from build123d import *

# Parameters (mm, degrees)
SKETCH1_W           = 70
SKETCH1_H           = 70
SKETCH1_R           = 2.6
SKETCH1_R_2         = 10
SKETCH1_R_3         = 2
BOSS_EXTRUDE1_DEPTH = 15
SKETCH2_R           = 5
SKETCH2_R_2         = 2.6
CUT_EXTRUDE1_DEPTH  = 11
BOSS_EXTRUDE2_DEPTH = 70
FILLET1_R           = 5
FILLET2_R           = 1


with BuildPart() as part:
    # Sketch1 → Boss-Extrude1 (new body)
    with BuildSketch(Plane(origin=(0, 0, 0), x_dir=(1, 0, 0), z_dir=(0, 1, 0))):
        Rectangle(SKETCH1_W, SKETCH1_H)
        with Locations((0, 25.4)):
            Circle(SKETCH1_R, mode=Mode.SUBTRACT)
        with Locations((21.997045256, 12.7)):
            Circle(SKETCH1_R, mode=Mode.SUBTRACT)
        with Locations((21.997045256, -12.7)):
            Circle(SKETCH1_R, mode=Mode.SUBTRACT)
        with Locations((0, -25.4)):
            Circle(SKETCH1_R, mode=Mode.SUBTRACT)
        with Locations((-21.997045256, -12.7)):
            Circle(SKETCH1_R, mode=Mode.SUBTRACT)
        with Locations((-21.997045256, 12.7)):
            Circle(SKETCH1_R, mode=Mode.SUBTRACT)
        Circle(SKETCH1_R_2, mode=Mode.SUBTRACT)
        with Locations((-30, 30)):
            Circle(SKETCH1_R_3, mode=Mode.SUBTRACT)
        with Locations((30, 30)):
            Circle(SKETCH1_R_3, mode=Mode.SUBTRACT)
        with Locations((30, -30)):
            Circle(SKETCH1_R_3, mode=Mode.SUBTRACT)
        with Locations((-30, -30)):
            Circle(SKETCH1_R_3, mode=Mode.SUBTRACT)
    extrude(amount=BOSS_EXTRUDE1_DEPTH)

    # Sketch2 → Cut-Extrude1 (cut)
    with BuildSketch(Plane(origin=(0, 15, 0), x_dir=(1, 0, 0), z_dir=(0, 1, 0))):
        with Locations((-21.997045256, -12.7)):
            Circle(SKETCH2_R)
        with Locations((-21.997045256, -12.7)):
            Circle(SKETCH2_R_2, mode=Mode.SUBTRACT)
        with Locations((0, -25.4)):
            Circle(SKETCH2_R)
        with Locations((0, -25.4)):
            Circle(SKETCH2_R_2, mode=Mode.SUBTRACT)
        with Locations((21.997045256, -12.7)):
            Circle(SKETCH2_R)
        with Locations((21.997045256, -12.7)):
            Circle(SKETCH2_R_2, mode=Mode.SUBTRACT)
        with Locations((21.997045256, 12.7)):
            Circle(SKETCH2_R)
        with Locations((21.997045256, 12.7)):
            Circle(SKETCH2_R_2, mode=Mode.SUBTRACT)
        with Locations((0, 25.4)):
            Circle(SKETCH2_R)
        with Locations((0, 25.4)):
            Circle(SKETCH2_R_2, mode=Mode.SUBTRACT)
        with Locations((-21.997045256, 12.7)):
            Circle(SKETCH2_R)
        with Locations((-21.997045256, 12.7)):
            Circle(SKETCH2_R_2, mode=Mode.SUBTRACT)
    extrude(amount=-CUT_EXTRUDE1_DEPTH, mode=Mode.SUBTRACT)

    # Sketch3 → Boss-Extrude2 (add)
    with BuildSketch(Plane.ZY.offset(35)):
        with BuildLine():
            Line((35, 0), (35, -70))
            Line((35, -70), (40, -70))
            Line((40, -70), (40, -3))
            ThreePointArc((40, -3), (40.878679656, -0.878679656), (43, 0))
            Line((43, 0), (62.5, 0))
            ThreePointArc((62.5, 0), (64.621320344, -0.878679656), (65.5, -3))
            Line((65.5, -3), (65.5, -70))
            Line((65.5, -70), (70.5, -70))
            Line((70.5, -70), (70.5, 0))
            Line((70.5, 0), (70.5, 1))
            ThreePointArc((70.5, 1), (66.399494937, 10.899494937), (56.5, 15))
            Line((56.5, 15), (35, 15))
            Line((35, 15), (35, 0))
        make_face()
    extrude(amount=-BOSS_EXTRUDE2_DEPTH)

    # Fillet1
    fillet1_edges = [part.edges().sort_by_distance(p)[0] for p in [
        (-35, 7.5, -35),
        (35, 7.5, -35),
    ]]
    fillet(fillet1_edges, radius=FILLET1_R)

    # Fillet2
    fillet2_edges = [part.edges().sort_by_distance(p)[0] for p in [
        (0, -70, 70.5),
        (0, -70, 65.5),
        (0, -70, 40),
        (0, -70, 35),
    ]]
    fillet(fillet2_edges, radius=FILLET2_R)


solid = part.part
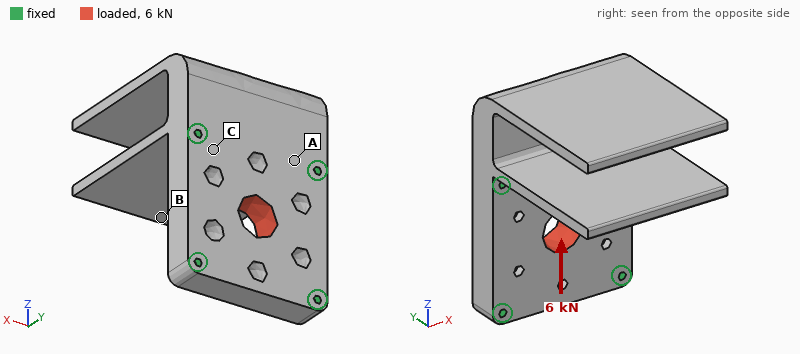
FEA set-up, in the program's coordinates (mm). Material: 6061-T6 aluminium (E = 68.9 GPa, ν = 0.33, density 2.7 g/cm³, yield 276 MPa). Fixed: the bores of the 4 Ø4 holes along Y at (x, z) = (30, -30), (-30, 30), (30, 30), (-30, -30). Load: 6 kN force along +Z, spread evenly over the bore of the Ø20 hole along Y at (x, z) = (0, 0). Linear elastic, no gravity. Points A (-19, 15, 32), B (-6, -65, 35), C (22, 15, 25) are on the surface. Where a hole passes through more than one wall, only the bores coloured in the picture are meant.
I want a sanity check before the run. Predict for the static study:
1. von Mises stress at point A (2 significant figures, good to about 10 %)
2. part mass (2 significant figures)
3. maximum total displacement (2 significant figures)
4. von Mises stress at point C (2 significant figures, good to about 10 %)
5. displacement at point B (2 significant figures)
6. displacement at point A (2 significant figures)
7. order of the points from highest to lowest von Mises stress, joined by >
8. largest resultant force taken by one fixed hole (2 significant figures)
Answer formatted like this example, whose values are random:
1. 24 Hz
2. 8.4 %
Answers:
1. 3.6 MPa
2. 390 g
3. 5.1 µm
4. 6.4 MPa
5. 2.8 µm
6. 1.5 µm
7. C > A > B
8. 1.8 kN
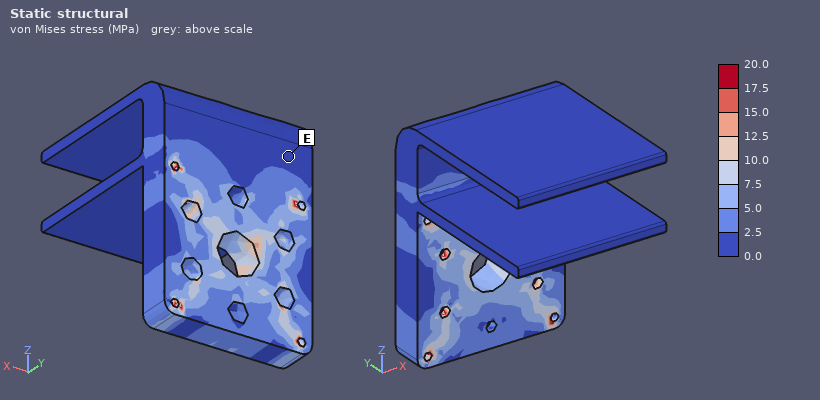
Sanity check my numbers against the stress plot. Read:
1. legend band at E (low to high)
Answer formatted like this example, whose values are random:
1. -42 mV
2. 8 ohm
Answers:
1. 0.0 to 2.5 MPa
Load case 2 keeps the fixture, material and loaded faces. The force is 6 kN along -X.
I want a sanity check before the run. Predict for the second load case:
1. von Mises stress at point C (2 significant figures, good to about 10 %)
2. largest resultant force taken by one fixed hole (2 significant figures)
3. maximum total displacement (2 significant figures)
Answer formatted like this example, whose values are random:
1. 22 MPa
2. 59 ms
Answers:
1. 9.4 MPa
2. 1.7 kN
3. 5.8 µm
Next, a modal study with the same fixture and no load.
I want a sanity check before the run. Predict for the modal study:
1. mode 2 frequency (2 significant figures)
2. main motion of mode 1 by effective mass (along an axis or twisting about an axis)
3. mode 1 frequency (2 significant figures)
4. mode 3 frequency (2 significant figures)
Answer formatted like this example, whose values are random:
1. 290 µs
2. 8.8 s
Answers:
1. 840 Hz
2. along Z
3. 780 Hz
4. 1900 Hz
